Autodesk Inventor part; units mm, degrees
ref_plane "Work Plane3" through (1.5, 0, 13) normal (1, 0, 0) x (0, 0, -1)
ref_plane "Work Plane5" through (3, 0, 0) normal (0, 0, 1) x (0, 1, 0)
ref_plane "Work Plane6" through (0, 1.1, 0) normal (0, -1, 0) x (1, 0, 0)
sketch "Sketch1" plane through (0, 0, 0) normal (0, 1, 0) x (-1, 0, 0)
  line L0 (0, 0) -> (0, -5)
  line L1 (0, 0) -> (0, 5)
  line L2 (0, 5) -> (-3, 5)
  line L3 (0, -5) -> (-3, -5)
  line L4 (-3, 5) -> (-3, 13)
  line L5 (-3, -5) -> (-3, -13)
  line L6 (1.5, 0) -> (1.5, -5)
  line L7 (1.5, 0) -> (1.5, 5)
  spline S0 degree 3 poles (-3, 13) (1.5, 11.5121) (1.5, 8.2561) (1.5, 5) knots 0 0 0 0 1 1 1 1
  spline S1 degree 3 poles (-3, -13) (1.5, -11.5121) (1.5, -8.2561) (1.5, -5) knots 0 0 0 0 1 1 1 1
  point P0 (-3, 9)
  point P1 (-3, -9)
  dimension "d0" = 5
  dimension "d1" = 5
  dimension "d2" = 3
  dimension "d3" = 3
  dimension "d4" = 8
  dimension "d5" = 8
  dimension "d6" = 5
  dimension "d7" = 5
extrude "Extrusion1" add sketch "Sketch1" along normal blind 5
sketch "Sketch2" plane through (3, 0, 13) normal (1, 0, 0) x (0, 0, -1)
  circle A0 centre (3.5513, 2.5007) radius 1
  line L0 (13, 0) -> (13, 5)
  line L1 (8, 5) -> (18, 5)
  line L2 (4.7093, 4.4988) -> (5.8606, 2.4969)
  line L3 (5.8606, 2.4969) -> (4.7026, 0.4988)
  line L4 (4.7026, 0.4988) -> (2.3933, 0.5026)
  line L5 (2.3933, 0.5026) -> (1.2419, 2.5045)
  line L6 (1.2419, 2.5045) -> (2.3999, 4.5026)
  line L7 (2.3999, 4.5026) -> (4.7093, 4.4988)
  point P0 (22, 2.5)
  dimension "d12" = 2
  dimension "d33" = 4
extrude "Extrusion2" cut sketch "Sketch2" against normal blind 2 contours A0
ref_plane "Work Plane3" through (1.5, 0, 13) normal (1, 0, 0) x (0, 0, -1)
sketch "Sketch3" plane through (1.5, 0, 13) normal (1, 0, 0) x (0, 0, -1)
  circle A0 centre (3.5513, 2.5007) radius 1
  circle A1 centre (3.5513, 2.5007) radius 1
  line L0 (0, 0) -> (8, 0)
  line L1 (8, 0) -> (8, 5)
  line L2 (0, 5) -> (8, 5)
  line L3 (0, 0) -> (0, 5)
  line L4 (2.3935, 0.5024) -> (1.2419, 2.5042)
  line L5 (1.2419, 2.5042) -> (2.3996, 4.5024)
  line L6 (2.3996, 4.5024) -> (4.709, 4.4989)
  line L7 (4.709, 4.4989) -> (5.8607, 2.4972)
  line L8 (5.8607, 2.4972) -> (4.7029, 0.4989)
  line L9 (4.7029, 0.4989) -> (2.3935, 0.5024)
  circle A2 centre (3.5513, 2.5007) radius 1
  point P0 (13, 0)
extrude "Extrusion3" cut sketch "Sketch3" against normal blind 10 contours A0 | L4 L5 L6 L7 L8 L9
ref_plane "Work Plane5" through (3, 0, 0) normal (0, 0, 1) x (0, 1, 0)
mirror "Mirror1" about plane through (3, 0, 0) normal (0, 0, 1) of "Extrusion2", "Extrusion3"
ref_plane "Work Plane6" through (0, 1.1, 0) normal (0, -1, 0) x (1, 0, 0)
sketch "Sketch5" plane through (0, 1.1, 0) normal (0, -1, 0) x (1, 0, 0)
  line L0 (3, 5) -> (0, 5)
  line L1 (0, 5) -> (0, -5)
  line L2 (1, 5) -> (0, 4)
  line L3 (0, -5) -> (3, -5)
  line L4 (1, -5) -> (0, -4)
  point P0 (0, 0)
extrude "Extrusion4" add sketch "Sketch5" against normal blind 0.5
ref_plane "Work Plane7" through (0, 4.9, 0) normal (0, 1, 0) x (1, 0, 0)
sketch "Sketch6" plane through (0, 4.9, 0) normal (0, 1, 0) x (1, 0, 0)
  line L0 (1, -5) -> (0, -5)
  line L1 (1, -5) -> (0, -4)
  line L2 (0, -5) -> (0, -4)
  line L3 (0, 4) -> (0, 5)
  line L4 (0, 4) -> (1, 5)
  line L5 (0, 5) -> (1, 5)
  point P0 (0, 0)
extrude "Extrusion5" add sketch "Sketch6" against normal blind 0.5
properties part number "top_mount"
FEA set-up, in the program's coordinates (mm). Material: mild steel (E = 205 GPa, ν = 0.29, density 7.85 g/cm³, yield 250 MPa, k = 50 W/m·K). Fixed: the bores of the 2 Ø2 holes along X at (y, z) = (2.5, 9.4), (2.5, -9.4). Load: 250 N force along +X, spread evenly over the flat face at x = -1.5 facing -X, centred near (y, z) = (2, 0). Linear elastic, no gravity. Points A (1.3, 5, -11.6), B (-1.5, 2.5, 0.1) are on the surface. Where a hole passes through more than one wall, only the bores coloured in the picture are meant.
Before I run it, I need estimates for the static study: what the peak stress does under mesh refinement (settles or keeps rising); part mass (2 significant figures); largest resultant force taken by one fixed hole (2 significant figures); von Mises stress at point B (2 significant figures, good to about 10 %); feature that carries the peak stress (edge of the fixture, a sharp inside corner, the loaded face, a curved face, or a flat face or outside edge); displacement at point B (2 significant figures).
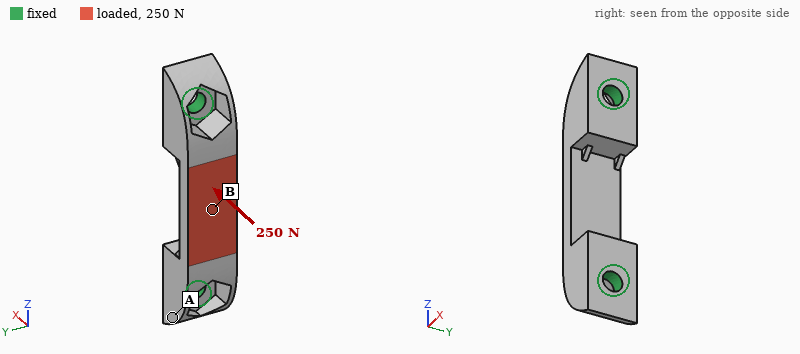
keeps rising
2.3 g
210 N
88 MPa
edge of the fixture
5.8 µm
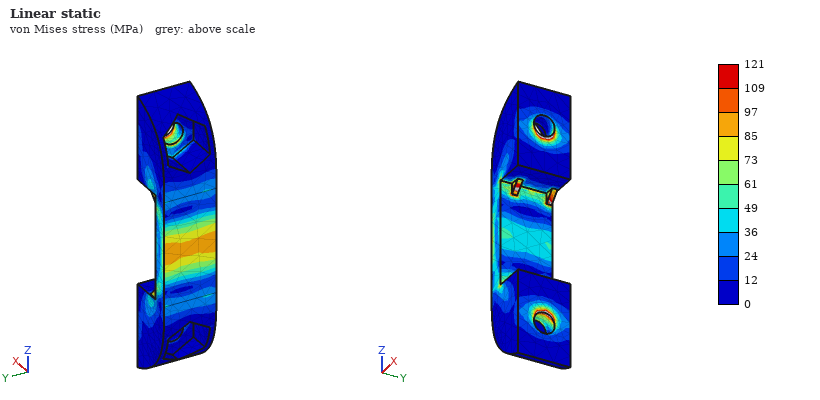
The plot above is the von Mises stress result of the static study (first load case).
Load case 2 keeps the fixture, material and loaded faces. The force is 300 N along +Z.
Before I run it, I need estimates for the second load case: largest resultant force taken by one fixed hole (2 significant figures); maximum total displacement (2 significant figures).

160 N
2.3 µm
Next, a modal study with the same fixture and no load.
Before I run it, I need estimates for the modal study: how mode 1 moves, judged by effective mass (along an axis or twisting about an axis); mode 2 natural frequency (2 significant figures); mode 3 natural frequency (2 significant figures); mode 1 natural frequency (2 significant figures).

along Y
44 kHz
45 kHz
35 kHz
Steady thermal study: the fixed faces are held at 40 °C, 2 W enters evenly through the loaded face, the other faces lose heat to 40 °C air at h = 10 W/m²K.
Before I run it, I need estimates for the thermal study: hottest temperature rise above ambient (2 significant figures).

16 K
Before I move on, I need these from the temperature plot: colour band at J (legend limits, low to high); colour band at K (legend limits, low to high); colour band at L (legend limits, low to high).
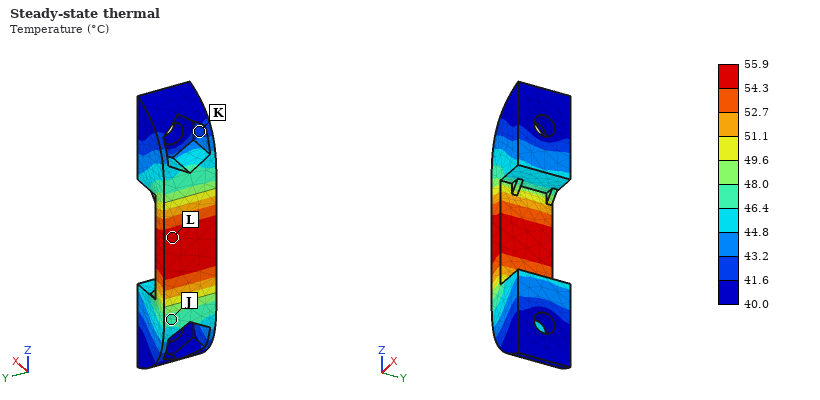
46.4 to 48.0 °C
41.6 to 43.2 °C
54.3 to 55.9 °C
